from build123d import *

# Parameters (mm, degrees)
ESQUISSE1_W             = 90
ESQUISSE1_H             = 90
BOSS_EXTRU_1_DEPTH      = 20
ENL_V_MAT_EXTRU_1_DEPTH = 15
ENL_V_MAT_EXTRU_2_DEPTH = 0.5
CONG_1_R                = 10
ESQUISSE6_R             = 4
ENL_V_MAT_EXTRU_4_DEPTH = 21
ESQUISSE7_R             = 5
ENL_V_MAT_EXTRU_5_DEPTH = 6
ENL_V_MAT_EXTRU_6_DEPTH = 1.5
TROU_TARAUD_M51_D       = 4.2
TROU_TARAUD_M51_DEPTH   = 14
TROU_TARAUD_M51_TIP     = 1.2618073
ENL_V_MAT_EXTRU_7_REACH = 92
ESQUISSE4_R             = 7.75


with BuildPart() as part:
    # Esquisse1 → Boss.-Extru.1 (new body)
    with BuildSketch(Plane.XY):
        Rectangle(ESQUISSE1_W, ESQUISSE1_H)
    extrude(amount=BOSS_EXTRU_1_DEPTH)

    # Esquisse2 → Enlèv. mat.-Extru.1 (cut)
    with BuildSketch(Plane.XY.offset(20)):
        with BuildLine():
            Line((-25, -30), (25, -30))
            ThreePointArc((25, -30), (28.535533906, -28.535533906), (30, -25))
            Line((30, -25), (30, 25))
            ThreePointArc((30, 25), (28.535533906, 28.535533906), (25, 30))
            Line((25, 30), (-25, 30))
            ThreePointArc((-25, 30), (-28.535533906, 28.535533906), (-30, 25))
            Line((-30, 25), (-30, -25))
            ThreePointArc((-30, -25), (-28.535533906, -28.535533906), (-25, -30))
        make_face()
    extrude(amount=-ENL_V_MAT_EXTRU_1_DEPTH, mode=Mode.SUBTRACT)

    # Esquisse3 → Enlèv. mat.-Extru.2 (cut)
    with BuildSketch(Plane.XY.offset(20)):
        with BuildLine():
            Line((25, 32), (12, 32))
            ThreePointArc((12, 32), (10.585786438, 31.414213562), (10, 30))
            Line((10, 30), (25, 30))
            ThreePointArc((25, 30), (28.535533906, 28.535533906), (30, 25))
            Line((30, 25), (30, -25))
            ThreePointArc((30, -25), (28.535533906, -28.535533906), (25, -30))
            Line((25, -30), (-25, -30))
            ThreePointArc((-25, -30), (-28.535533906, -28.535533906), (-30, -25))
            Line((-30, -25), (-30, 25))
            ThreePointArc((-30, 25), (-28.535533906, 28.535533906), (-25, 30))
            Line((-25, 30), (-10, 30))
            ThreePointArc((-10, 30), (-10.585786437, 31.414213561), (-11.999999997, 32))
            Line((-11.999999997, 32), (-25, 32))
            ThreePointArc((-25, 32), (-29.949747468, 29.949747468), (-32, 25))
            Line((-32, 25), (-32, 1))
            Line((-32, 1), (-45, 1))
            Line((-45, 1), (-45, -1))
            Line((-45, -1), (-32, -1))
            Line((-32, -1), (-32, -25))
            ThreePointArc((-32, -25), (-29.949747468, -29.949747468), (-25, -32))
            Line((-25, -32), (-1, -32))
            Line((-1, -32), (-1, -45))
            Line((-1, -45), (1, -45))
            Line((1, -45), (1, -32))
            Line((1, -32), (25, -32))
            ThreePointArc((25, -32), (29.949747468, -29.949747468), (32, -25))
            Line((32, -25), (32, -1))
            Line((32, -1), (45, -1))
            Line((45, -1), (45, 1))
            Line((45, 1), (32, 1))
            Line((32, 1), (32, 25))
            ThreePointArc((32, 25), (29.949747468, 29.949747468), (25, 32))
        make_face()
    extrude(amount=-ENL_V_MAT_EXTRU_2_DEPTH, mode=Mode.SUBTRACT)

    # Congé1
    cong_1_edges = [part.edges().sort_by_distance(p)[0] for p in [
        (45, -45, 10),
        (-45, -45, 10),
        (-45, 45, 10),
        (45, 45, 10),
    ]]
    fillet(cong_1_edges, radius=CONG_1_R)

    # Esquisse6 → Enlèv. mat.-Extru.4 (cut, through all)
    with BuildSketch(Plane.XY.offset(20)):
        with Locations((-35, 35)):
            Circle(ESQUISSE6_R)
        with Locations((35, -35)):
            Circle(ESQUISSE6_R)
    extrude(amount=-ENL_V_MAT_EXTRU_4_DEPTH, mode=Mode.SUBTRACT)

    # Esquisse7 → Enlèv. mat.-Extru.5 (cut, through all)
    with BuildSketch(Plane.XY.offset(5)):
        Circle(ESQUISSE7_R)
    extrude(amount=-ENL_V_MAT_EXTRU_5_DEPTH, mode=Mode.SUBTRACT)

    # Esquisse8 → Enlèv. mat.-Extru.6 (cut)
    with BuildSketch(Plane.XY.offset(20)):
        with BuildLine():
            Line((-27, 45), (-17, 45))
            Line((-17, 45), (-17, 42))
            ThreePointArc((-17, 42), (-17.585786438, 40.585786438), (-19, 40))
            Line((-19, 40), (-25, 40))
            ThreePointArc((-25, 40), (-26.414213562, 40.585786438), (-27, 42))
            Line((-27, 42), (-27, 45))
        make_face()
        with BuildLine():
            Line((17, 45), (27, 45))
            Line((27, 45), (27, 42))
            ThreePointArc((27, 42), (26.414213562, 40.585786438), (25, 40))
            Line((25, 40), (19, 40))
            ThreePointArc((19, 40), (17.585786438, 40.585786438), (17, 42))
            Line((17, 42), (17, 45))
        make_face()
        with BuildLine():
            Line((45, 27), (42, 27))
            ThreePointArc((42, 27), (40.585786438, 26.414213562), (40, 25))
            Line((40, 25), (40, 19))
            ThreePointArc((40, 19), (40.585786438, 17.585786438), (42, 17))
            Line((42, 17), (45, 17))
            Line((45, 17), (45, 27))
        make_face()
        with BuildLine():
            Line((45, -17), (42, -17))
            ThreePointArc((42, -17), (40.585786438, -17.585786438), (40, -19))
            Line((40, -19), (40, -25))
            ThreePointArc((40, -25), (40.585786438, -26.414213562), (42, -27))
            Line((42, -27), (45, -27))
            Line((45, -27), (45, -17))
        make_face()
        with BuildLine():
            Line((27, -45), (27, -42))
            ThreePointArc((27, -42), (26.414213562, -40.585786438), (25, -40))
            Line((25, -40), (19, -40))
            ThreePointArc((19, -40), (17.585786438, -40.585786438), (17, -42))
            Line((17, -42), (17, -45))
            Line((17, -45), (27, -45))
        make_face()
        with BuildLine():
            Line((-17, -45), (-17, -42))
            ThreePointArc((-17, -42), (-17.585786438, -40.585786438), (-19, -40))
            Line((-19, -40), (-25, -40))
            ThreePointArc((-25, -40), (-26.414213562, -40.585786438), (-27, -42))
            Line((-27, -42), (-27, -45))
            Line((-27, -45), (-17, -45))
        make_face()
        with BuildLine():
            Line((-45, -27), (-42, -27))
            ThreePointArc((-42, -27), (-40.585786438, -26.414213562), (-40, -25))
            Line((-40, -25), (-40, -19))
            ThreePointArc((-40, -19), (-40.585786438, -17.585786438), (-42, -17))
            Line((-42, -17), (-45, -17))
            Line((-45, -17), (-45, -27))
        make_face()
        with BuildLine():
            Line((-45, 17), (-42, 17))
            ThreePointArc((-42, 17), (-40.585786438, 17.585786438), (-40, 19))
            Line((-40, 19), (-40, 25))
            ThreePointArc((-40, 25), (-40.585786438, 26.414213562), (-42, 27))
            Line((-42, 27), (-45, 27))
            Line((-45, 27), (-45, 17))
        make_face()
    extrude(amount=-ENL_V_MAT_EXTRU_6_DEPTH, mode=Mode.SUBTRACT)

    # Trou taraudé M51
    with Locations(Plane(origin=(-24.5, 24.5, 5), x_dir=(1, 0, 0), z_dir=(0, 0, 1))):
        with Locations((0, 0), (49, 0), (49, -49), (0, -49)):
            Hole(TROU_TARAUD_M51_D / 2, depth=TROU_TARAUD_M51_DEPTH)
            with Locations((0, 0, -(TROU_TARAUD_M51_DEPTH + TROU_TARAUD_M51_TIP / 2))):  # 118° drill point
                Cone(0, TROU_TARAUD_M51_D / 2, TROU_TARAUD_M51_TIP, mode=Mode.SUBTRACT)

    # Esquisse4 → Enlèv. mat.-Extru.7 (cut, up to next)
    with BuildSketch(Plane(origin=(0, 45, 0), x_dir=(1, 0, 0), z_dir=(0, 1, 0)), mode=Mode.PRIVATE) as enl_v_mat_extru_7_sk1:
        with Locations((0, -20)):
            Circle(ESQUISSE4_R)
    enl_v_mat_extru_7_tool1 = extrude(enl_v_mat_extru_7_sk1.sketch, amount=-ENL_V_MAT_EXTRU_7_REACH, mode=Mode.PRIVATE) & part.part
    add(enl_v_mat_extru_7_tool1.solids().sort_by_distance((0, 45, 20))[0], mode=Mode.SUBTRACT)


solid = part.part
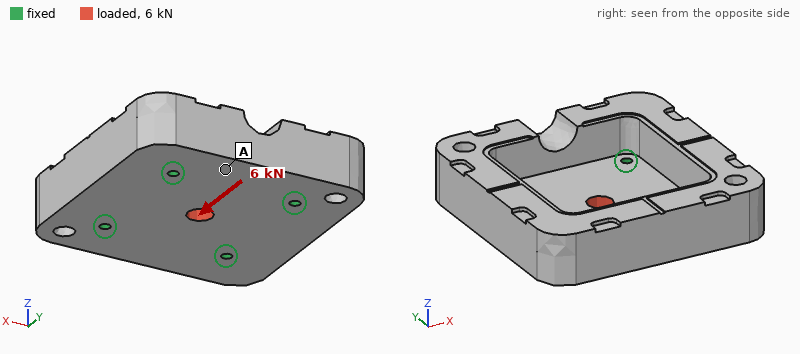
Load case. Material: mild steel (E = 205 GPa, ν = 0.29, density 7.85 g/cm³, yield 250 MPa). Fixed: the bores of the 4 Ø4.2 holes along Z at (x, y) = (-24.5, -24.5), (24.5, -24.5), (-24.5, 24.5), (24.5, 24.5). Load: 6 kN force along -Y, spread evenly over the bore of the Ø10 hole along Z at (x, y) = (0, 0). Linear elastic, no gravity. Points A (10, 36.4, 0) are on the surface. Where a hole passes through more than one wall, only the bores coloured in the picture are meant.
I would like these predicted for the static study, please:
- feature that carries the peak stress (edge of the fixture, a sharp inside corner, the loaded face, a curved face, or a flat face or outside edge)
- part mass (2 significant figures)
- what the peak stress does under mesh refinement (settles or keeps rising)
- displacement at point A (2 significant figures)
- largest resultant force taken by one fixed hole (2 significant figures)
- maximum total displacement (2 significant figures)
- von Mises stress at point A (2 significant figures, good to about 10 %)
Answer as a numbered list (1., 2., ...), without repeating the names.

1. a sharp inside corner
2. 800 g
3. keeps rising
4. 1.3 µm
5. 1.6 kN
6. 3.8 µm
7. 7.3 MPa
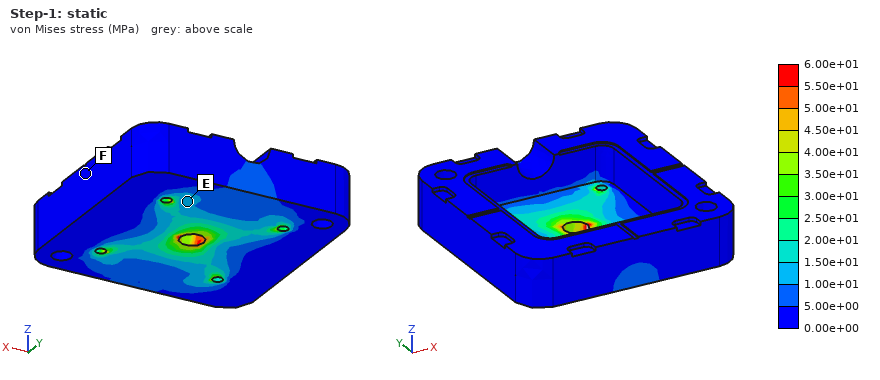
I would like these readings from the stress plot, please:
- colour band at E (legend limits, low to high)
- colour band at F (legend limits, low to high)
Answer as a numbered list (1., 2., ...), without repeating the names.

1. 1.00e+01 to 1.50e+01 MPa
2. 0.00e+00 to 5.00e+00 MPa
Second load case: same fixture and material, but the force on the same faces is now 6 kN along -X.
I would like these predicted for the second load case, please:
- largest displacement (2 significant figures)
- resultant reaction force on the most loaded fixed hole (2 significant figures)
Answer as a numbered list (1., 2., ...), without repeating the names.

1. 3.8 µm
2. 1.6 kN
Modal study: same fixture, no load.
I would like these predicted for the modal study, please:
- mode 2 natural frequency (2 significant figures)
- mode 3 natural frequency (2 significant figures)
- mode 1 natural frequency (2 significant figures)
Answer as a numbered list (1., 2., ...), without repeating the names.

1. 6800 Hz
2. 7000 Hz
3. 6700 Hz
